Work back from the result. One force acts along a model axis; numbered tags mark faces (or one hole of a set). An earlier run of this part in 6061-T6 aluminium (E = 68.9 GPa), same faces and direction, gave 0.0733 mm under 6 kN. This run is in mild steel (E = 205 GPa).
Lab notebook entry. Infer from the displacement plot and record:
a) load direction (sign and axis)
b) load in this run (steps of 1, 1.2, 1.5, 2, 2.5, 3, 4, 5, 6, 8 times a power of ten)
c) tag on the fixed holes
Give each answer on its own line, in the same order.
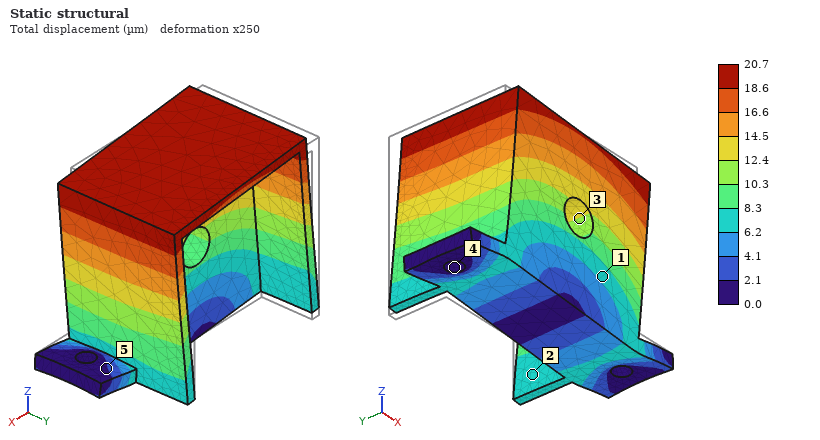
+X
5 kN
4
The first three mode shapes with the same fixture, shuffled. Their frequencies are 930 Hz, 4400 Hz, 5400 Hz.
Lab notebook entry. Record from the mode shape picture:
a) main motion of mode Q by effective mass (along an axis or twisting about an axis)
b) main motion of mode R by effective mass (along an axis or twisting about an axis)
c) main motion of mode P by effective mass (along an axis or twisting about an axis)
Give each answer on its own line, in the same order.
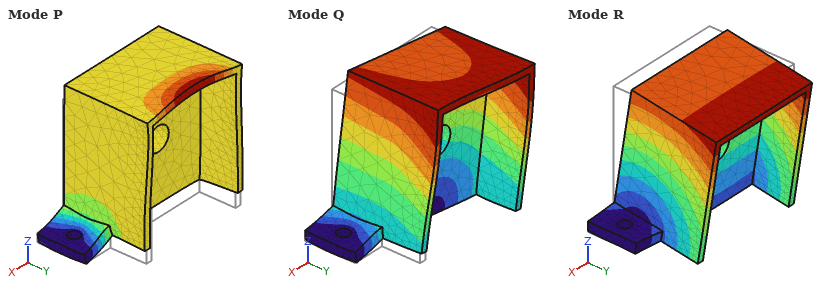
along X
along Y
along Z
